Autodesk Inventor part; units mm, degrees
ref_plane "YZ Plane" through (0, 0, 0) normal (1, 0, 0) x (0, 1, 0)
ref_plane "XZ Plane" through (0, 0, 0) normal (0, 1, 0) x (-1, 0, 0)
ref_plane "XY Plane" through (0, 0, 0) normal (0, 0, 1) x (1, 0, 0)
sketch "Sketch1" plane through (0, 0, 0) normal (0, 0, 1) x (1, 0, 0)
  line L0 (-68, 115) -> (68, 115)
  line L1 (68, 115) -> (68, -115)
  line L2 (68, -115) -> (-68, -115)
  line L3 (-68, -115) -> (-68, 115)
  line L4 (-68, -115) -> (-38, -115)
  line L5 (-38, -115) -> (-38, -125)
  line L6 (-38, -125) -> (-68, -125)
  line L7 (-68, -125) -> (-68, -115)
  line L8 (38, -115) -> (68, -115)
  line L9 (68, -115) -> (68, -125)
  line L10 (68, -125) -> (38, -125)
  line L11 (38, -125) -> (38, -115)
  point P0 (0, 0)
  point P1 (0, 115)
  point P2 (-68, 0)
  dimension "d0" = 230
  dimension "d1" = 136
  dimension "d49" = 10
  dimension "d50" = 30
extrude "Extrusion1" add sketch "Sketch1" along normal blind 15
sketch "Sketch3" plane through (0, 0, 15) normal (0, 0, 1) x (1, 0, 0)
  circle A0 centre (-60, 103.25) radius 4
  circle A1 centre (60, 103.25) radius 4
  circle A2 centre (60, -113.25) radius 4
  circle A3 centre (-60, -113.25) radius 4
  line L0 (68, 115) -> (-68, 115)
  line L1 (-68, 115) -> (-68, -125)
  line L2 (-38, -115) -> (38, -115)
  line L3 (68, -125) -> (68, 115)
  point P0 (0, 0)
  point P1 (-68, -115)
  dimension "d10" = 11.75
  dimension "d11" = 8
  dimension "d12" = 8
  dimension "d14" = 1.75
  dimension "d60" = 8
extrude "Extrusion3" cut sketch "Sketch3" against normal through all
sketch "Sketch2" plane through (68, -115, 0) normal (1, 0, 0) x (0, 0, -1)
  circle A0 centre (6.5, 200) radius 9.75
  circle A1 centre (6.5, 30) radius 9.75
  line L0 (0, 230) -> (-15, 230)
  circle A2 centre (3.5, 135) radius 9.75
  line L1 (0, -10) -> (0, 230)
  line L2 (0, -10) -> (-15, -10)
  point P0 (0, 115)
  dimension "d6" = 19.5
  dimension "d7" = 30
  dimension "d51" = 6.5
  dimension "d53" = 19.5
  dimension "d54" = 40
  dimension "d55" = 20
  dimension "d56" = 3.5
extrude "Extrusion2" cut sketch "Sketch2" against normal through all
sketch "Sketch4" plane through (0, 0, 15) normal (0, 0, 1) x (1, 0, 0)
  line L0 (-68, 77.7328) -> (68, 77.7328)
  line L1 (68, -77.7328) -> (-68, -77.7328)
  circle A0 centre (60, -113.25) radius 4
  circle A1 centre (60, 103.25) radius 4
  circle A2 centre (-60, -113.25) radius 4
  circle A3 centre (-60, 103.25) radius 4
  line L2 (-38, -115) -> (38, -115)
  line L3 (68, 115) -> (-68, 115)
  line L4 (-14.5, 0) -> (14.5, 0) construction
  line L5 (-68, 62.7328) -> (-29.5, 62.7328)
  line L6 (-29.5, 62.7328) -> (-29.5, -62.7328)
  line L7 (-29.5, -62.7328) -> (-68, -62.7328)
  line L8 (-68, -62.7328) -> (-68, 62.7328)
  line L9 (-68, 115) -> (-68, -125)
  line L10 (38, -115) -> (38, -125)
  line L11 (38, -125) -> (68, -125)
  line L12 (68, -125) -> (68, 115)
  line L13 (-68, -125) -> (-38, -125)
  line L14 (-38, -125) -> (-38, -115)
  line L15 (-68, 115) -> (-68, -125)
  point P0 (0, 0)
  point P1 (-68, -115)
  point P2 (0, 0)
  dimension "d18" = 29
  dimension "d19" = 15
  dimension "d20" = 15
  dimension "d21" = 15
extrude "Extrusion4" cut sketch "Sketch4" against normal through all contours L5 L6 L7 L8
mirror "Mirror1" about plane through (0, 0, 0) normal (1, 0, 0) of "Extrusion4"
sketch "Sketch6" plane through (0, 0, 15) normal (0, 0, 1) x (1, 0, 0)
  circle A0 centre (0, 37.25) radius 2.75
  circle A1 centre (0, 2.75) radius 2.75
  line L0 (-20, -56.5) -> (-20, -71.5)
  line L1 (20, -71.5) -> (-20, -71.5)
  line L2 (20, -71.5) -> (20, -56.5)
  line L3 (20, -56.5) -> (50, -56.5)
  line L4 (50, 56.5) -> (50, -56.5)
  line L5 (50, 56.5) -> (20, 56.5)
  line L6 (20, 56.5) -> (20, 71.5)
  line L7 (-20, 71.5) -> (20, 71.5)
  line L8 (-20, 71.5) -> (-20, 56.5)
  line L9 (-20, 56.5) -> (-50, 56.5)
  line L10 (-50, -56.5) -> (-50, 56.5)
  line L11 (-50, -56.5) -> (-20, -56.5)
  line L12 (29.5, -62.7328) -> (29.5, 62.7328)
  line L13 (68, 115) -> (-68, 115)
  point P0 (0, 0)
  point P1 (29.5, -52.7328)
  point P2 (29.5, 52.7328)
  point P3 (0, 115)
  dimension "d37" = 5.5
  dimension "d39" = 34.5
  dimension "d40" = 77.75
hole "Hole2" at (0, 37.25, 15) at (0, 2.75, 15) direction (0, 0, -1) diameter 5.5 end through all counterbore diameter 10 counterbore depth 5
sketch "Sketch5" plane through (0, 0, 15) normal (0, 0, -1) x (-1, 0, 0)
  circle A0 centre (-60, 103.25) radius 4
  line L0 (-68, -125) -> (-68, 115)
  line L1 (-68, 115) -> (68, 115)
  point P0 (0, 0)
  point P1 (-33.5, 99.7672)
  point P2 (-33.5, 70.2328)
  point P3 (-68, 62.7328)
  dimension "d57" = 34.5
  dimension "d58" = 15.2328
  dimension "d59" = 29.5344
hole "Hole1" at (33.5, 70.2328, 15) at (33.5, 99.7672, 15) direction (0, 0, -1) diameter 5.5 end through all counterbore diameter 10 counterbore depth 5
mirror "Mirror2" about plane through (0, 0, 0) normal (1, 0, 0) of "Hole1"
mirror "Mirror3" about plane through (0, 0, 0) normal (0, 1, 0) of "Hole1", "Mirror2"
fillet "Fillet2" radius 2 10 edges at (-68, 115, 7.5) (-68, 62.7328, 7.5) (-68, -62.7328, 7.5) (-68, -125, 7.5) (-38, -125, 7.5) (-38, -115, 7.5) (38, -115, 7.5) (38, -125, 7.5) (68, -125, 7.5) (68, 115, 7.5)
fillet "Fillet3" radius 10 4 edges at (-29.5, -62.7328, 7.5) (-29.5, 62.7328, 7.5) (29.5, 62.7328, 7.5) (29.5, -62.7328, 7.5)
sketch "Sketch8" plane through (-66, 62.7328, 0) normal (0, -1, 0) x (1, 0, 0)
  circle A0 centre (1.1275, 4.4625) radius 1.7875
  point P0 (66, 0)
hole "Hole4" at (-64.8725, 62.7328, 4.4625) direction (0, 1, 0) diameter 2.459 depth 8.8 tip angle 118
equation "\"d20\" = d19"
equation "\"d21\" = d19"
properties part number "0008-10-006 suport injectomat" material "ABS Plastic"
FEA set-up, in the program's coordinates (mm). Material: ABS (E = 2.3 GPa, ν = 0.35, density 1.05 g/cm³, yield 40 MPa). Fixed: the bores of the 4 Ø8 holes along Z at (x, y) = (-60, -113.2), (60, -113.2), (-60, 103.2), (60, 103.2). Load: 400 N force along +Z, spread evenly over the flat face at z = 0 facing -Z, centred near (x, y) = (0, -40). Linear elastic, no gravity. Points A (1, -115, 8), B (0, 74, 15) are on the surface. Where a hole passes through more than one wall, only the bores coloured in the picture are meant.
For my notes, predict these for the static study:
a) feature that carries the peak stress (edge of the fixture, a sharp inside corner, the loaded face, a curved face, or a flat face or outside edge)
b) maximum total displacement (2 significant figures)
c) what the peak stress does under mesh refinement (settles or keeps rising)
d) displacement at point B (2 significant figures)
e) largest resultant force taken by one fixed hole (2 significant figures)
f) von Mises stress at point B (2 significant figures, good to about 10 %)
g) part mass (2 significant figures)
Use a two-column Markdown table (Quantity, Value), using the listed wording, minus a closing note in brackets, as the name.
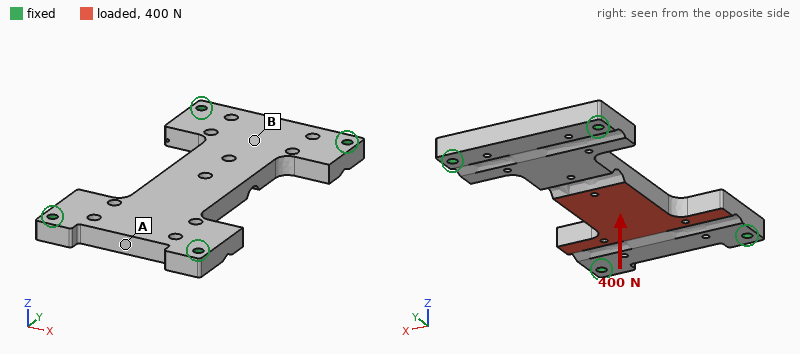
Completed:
| Quantity | Value |
|---|---|
| feature that carries the peak stress | edge of the fixture |
| maximum total displacement | 0.56 mm |
| what the peak stress does under mesh refinement | keeps rising |
| displacement at point B | 0.16 mm |
| largest resultant force taken by one fixed hole | 140 N |
| von Mises stress at point B | 1.1 MPa |
| part mass | 330 g |
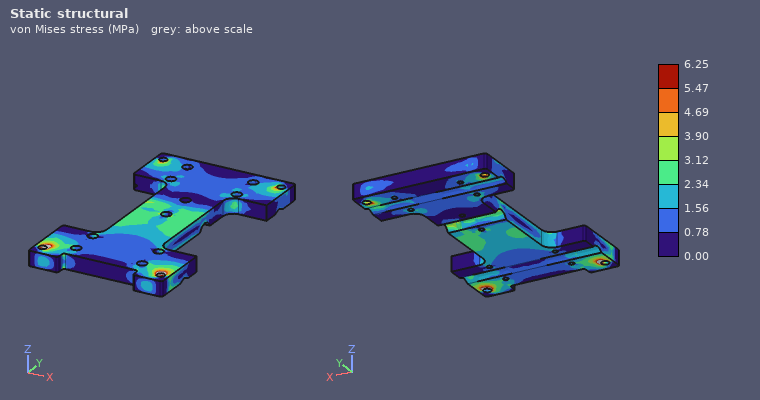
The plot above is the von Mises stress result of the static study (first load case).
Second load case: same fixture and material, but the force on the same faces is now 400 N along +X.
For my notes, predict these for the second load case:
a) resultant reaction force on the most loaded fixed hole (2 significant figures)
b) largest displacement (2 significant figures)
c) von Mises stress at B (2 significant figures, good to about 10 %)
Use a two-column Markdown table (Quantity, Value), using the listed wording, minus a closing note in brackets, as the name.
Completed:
| Quantity | Value |
|---|---|
| resultant reaction force on the most loaded fixed hole | 210 N |
| largest displacement | 56 µm |
| von Mises stress at B | 0.13 MPa |
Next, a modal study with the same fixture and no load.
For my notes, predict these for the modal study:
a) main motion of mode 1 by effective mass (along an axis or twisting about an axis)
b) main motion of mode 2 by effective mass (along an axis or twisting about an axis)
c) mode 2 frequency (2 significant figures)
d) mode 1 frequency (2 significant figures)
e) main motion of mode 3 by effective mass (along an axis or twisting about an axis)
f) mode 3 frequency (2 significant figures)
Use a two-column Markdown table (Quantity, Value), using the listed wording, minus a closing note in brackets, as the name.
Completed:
| Quantity | Value |
|---|---|
| main motion of mode 1 by effective mass | along Z |
| main motion of mode 2 by effective mass | twisting about X |
| mode 2 frequency | 900 Hz |
| mode 1 frequency | 380 Hz |
| main motion of mode 3 by effective mass | twisting about Y |
| mode 3 frequency | 1100 Hz |
